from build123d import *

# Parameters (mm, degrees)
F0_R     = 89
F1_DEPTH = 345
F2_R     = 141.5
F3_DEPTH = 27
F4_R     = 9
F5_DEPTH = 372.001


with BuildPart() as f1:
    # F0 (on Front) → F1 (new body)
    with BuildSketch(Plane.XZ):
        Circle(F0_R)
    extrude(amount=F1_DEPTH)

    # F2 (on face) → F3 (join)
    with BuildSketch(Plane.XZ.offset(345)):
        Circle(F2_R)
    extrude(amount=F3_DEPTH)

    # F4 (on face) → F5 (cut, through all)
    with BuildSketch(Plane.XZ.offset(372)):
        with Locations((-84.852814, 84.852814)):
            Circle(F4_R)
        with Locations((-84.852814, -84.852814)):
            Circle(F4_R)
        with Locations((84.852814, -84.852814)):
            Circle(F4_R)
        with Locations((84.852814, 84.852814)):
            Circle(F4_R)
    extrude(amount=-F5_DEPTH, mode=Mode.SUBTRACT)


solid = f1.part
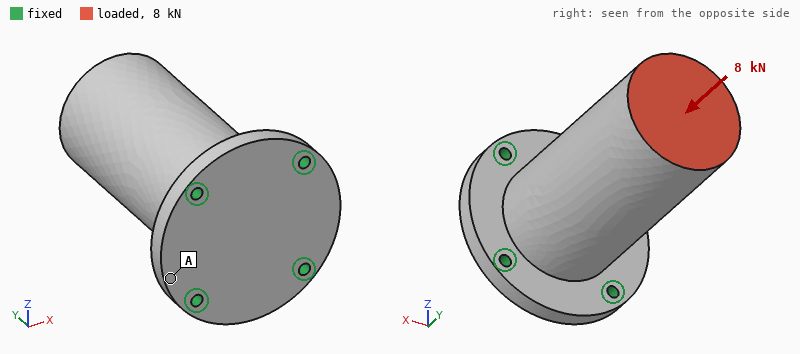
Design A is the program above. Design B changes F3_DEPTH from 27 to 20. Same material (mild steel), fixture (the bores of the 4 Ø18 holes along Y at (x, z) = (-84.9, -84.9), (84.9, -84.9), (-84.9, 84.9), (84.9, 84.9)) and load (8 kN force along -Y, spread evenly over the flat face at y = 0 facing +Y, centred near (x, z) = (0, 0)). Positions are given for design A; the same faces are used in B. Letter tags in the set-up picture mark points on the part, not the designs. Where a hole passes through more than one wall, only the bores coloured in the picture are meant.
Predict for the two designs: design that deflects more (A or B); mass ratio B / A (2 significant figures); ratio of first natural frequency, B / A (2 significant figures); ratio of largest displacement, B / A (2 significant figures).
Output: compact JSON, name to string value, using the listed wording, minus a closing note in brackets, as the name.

{"design that deflects more": "B", "mass ratio B / A": "0.96", "ratio of first natural frequency, B / A": "0.83", "ratio of largest displacement, B / A": "1.4"}
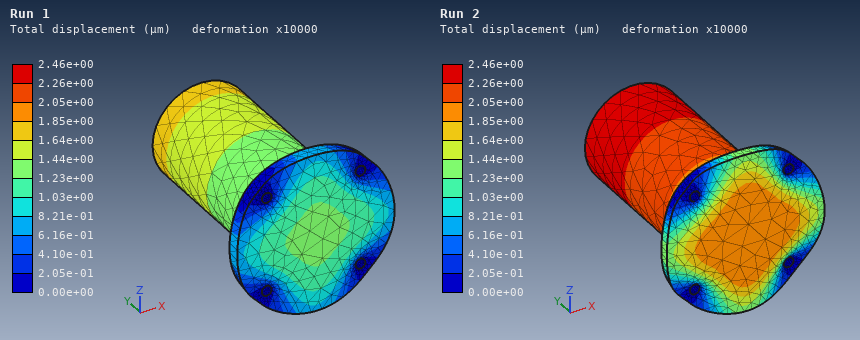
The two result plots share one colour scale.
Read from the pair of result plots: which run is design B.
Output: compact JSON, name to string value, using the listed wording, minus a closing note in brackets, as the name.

{"which run is design B": "Run 2"}
